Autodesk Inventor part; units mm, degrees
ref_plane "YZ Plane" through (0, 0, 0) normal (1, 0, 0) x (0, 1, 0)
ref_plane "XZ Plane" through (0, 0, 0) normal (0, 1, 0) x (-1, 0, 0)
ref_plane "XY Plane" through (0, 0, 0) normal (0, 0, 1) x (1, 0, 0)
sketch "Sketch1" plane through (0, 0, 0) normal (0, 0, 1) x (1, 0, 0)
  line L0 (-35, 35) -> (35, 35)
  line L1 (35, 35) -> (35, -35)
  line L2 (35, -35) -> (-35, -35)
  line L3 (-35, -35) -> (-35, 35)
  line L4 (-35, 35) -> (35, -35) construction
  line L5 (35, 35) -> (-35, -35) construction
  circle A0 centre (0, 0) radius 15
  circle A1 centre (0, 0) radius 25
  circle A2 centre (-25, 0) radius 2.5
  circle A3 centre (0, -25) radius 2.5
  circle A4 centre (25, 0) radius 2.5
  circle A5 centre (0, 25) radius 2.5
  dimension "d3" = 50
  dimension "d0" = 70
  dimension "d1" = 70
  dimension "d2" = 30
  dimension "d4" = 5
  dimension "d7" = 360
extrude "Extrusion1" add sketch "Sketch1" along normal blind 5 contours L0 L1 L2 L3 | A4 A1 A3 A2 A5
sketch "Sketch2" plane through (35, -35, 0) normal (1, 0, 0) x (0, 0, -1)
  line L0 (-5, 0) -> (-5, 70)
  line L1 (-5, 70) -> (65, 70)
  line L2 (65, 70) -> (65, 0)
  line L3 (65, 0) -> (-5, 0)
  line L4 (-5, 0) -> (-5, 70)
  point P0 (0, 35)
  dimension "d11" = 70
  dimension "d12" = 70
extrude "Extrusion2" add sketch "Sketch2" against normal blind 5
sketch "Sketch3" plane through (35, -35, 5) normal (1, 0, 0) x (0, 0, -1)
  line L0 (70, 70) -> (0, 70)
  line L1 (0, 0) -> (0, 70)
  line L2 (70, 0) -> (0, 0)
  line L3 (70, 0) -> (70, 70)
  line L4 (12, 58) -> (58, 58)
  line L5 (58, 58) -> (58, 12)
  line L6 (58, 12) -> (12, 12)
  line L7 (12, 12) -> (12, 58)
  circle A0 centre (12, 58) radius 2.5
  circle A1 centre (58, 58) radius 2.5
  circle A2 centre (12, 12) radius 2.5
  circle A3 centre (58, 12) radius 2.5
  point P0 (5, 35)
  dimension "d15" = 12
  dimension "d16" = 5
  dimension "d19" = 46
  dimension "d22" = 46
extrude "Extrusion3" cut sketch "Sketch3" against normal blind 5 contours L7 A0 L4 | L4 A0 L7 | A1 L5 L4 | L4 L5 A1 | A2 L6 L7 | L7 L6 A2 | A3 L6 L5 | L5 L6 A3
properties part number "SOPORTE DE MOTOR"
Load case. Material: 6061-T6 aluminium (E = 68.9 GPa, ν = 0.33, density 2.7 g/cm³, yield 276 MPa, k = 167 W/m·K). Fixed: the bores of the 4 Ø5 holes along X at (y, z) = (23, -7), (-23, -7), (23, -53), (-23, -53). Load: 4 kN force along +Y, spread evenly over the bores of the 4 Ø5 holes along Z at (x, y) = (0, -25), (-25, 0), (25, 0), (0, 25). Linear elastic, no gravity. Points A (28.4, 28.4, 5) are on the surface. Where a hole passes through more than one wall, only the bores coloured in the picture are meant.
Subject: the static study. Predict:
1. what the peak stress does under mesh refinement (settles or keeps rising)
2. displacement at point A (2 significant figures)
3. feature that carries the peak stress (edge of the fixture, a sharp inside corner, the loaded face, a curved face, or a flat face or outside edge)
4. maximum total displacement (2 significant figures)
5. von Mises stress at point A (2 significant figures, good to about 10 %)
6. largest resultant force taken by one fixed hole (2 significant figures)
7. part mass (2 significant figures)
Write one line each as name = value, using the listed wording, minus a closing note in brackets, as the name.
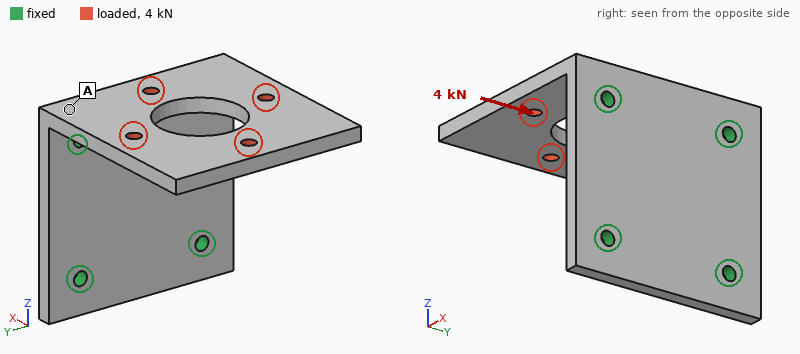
what the peak stress does under mesh refinement = keeps rising
displacement at point A = 0.062 mm
feature that carries the peak stress = edge of the fixture
maximum total displacement = 0.23 mm
von Mises stress at point A = 35 MPa
largest resultant force taken by one fixed hole = 3.4 kN
part mass = 120 g
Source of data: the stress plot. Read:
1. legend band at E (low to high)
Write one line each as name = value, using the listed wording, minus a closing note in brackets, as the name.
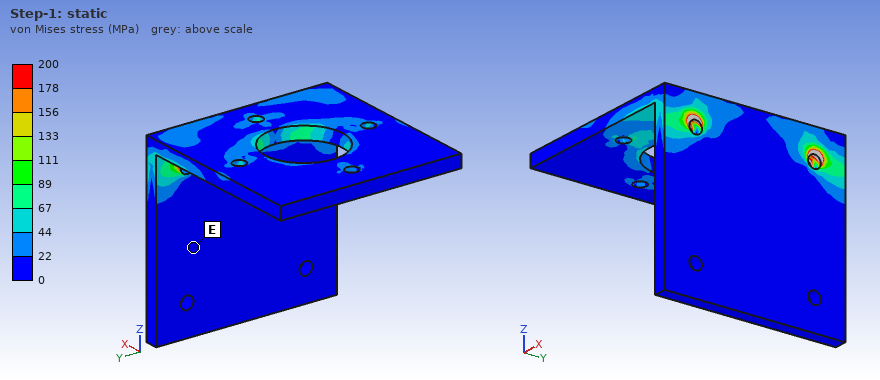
legend band at E = 0 to 22 MPa
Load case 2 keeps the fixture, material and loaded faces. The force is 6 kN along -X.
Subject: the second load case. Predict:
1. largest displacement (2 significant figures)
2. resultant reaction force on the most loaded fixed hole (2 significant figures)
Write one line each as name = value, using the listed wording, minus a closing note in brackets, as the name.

largest displacement = 0.45 mm
resultant reaction force on the most loaded fixed hole = 3.1 kN
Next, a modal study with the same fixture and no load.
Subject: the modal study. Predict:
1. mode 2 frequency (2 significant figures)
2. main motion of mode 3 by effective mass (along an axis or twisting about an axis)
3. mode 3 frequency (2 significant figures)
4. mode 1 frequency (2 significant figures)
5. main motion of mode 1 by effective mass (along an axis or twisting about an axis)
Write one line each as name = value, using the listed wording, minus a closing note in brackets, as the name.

mode 2 frequency = 1700 Hz
main motion of mode 3 by effective mass = along Y
mode 3 frequency = 3600 Hz
mode 1 frequency = 710 Hz
main motion of mode 1 by effective mass = along Z
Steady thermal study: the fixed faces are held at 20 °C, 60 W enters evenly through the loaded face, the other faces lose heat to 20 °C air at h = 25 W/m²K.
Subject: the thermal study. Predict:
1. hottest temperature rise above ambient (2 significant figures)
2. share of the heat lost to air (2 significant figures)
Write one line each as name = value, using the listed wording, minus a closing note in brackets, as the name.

hottest temperature rise above ambient = 55 K
share of the heat lost to air = 15 %
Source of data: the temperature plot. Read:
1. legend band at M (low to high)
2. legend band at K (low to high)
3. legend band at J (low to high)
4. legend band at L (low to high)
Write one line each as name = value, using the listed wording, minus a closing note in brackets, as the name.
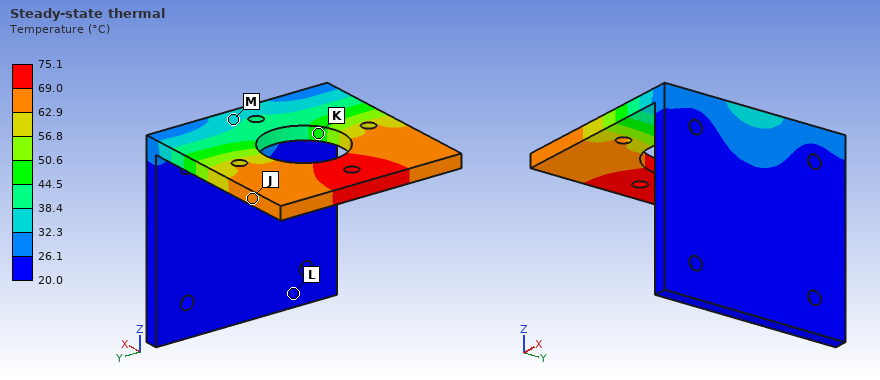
legend band at M = 32.3 to 38.4 °C
legend band at K = 44.5 to 50.6 °C
legend band at J = 62.9 to 69.0 °C
legend band at L = 20.0 to 26.1 °C
